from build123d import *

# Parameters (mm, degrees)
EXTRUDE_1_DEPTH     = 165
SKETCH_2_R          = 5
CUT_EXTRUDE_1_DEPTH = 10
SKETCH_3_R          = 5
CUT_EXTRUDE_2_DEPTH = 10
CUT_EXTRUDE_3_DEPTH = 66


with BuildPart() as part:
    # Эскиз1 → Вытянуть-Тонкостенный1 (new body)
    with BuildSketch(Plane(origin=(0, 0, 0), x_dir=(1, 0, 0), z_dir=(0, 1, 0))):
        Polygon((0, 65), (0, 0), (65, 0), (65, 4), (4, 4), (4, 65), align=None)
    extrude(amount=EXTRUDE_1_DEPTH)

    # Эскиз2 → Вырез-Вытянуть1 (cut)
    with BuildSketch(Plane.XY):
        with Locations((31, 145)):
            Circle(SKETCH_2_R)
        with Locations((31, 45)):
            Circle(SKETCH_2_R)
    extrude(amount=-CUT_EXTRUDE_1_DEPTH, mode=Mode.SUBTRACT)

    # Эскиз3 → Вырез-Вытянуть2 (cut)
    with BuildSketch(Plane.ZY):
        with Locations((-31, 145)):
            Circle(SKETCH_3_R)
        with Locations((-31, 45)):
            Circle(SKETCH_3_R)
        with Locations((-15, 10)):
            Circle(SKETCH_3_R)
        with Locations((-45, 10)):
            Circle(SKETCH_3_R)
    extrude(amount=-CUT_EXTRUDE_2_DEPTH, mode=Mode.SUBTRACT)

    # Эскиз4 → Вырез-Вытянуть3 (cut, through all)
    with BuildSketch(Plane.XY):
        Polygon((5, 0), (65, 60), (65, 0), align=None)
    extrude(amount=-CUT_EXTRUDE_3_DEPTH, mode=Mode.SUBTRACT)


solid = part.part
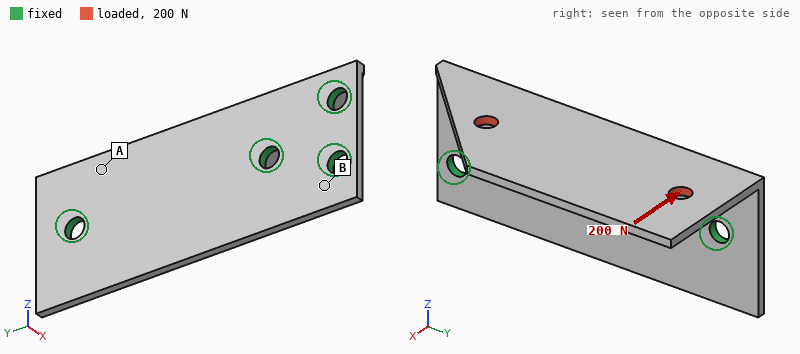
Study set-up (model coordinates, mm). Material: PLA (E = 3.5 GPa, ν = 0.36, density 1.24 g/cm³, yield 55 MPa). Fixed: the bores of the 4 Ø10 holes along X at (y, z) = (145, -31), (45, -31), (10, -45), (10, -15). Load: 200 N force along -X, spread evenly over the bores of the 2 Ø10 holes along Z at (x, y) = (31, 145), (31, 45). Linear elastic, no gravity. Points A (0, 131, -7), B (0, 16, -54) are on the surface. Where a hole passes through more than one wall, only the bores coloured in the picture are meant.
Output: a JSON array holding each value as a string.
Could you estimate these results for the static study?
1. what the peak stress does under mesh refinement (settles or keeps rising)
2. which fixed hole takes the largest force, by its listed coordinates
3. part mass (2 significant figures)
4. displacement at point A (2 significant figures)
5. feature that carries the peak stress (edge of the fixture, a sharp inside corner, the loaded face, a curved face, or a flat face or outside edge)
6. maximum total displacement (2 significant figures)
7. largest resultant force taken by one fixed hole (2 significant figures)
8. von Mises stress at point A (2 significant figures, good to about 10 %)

["keeps rising", "(145, -31)", "92 g", "0.47 mm", "edge of the fixture", "2.0 mm", "120 N", "4.6 MPa"]
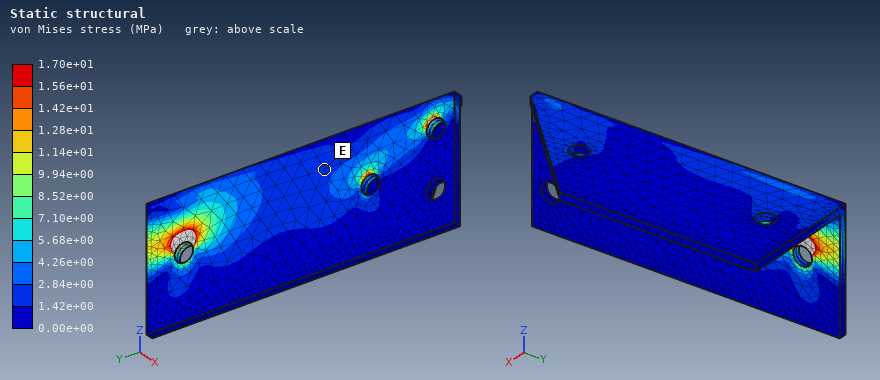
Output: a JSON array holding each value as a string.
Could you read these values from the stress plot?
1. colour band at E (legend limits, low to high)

["1.42e+00 to 2.84e+00 MPa"]
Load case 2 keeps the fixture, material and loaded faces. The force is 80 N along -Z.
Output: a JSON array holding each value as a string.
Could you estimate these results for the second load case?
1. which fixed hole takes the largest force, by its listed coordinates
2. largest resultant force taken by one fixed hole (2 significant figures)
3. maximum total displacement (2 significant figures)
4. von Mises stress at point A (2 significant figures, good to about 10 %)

["(45, -31)", "52 N", "2.1 mm", "5.2 MPa"]
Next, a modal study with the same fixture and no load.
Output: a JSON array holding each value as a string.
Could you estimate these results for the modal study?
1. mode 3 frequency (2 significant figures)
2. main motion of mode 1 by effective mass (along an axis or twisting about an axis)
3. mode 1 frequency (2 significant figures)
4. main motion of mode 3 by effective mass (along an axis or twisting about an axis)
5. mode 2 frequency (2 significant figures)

["550 Hz", "along Z", "180 Hz", "along X", "420 Hz"]
